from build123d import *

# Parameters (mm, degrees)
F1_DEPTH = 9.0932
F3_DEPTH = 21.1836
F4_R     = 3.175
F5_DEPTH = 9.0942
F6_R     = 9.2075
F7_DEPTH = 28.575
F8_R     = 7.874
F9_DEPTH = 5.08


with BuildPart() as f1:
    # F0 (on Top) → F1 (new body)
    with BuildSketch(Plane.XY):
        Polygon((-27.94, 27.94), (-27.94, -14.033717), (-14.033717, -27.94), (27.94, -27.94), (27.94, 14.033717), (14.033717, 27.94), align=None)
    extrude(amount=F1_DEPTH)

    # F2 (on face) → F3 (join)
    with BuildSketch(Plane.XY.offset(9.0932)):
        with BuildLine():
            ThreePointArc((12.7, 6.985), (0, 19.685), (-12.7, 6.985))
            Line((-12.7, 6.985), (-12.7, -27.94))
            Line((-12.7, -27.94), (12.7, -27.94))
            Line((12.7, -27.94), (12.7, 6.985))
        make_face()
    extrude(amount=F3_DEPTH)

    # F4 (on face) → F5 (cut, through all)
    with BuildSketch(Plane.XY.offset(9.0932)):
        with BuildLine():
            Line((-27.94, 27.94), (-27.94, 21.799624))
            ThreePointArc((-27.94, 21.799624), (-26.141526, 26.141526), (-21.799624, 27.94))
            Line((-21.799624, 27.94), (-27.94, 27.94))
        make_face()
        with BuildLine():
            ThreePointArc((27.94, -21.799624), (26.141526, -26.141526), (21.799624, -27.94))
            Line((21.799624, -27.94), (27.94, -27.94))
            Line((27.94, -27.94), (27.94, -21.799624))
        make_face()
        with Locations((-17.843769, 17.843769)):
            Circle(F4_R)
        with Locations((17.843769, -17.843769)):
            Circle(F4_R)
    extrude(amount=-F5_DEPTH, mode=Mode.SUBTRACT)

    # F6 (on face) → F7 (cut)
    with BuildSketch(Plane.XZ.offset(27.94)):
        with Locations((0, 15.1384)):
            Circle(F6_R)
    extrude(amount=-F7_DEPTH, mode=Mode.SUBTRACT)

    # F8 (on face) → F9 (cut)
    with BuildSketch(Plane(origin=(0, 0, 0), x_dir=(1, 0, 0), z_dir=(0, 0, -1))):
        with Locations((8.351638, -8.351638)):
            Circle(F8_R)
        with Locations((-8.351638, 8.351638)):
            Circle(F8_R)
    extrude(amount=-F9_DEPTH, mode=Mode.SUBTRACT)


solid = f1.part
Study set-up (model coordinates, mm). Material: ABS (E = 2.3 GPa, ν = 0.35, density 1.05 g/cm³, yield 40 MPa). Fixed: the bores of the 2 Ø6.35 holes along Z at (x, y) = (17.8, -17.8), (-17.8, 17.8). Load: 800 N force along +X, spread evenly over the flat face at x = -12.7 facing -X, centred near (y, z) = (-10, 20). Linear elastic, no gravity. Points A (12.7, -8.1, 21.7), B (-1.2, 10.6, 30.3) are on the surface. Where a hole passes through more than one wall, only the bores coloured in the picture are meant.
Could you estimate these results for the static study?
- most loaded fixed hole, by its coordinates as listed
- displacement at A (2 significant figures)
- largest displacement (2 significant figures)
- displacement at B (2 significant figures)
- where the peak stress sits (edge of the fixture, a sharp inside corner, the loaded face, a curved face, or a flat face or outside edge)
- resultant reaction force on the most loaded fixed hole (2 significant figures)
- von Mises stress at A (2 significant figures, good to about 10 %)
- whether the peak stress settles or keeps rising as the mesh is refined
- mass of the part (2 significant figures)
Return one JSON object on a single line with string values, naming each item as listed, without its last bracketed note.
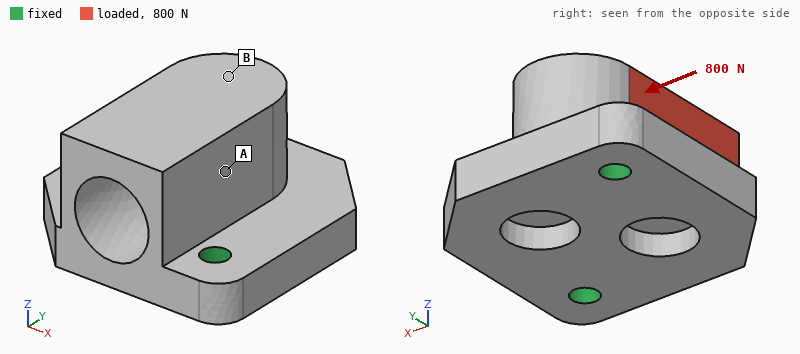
{"most loaded fixed hole, by its coordinates as listed": "(17.8, -17.8)", "displacement at A": "0.25 mm", "largest displacement": "0.44 mm", "displacement at B": "0.29 mm", "where the peak stress sits": "edge of the fixture", "resultant reaction force on the most loaded fixed hole": "540 N", "von Mises stress at A": "3.8 MPa", "whether the peak stress settles or keeps rising as the mesh is refined": "keeps rising", "mass of the part": "43 g"}
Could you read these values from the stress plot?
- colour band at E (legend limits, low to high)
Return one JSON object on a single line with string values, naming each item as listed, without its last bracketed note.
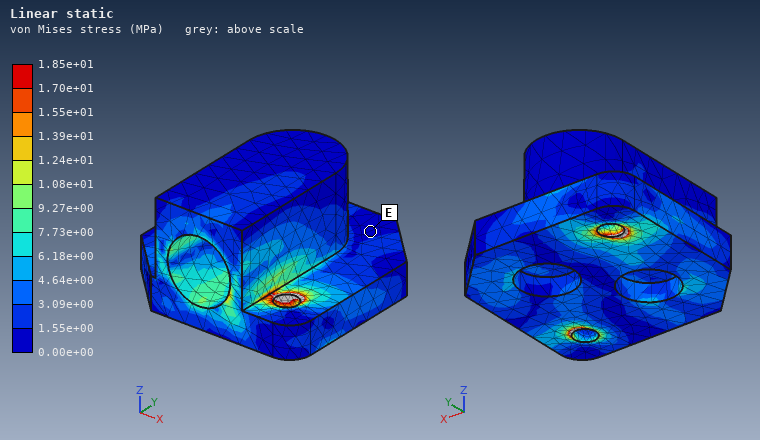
{"colour band at E": "0.00e+00 to 1.55e+00 MPa"}
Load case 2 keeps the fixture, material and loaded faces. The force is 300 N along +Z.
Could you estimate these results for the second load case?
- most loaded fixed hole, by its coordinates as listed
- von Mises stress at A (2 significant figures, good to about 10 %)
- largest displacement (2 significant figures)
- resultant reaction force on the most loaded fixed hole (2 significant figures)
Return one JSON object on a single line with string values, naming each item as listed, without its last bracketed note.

{"most loaded fixed hole, by its coordinates as listed": "(-17.8, 17.8)", "von Mises stress at A": "1.4 MPa", "largest displacement": "0.24 mm", "resultant reaction force on the most loaded fixed hole": "190 N"}
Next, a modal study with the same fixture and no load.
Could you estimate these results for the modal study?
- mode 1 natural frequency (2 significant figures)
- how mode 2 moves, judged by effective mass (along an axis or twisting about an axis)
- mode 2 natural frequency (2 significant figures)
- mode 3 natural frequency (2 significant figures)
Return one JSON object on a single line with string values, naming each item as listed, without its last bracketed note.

{"mode 1 natural frequency": "1400 Hz", "how mode 2 moves, judged by effective mass": "along Z", "mode 2 natural frequency": "3000 Hz", "mode 3 natural frequency": "3500 Hz"}
